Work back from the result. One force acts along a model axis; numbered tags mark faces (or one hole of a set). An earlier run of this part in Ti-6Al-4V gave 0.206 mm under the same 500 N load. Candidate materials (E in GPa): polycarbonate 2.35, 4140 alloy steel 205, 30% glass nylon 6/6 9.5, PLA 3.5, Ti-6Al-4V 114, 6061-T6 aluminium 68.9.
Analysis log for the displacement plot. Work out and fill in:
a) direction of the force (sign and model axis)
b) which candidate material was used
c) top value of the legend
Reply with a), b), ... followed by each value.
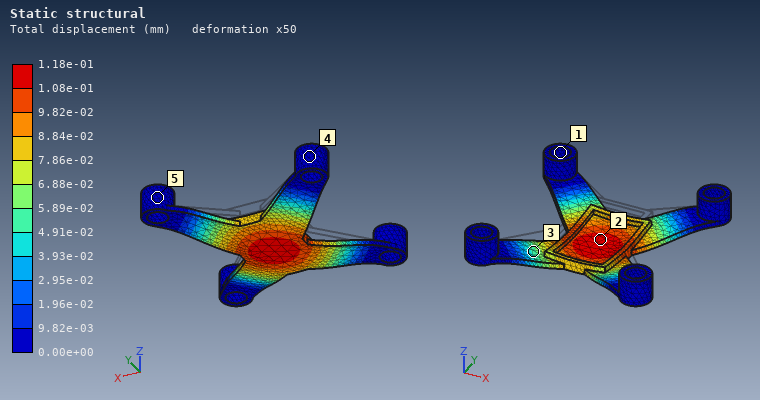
a) -Z
b) 4140 alloy steel
c) 1.18e-01 mm
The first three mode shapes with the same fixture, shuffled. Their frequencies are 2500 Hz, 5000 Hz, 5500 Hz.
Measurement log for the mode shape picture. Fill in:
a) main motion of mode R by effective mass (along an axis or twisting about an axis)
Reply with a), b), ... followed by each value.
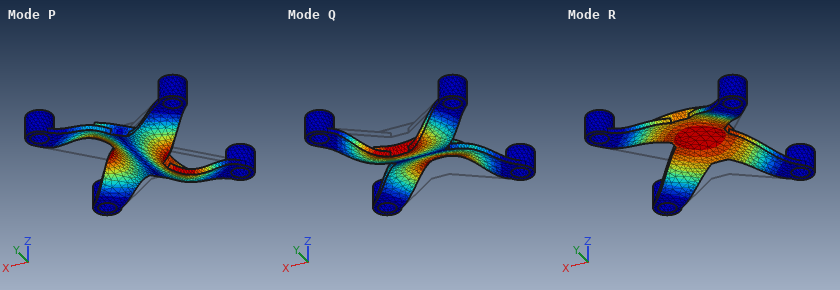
a) along Z
